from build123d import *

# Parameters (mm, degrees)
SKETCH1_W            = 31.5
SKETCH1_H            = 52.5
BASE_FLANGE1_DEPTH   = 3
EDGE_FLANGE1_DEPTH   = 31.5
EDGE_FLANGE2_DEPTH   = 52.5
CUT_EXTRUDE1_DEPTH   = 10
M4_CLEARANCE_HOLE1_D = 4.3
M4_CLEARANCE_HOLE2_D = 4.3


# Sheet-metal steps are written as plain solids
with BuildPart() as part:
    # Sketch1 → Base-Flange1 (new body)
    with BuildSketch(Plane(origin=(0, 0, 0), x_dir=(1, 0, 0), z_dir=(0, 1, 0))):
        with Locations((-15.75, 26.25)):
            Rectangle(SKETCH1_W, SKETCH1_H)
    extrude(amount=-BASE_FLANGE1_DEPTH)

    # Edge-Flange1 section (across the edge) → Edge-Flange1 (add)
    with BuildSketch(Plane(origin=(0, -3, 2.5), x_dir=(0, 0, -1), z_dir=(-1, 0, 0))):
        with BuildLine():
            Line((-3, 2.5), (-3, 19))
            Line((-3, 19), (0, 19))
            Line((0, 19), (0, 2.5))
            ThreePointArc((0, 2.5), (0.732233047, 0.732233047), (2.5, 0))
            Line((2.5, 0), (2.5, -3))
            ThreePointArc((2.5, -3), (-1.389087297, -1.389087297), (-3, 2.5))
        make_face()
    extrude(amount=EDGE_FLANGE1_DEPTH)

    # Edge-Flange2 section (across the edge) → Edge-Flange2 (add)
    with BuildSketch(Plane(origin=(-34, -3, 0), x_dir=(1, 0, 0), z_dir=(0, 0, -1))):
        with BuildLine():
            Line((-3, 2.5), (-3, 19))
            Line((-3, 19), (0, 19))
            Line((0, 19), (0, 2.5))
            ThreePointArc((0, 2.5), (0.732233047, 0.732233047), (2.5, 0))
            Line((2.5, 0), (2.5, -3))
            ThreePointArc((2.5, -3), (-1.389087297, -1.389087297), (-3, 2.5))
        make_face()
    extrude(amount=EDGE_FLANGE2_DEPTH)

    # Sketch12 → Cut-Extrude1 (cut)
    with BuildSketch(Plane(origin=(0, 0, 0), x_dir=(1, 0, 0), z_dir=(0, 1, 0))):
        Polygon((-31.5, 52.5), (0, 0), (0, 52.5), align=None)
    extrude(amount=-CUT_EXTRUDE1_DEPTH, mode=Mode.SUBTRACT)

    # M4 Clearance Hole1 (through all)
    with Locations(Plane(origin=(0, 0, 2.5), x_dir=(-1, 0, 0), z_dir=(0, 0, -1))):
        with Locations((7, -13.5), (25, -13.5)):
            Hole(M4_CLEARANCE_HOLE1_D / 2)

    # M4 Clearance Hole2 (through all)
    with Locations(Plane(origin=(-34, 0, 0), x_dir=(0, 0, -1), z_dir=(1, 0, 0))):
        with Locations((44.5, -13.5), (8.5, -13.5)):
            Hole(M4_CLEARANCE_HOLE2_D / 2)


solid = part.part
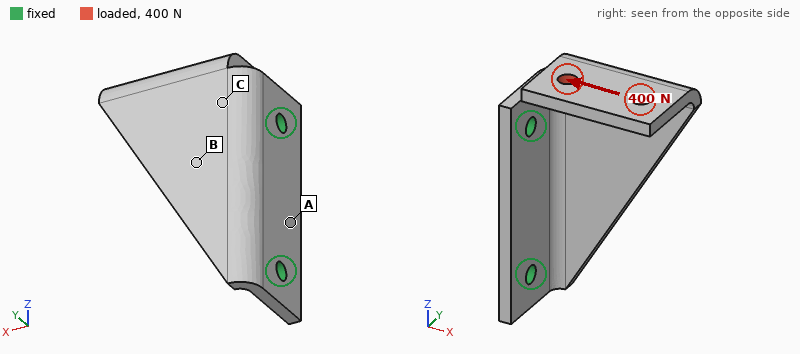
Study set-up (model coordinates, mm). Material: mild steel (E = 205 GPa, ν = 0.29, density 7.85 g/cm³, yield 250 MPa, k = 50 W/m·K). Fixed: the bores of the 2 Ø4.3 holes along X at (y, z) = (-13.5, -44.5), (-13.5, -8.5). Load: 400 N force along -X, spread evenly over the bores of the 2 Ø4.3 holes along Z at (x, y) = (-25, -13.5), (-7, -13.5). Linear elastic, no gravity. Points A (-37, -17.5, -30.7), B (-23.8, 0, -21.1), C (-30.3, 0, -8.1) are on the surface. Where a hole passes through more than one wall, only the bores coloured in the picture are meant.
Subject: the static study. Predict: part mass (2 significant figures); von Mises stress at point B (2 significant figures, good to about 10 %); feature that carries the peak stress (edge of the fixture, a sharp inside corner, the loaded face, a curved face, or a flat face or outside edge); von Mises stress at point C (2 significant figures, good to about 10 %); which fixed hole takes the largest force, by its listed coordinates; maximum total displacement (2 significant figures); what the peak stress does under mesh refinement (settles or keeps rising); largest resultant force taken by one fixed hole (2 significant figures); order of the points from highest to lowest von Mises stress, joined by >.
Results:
63 g
56 MPa
a sharp inside corner
98 MPa
(-13.5, -8.5)
0.23 mm
keeps rising
520 N
C > B > A
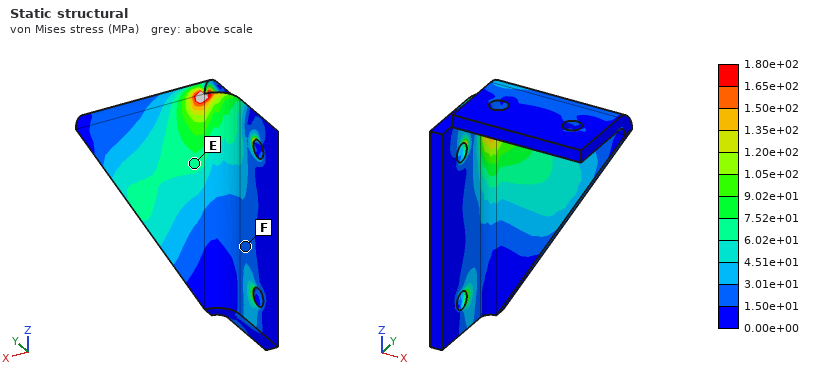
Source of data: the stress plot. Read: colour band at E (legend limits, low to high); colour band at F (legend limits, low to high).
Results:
6.02e+01 to 7.52e+01 MPa
1.50e+01 to 3.01e+01 MPa
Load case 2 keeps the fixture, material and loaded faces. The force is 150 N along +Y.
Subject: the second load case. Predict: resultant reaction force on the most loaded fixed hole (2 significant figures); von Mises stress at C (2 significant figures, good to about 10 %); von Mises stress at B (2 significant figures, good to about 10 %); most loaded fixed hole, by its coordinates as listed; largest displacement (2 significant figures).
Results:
200 N
59 MPa
39 MPa
(-13.5, -8.5)
0.19 mm
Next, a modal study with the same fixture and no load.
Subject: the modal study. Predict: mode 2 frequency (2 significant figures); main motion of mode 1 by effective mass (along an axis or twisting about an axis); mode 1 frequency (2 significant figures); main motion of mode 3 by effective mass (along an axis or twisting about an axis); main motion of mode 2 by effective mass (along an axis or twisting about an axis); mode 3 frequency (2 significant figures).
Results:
2600 Hz
along Y
1200 Hz
along X
along Z
3600 Hz
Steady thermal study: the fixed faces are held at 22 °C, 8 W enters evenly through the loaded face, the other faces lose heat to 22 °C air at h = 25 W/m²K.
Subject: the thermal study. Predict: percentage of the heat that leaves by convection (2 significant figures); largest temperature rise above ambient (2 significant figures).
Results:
41 %
61 K
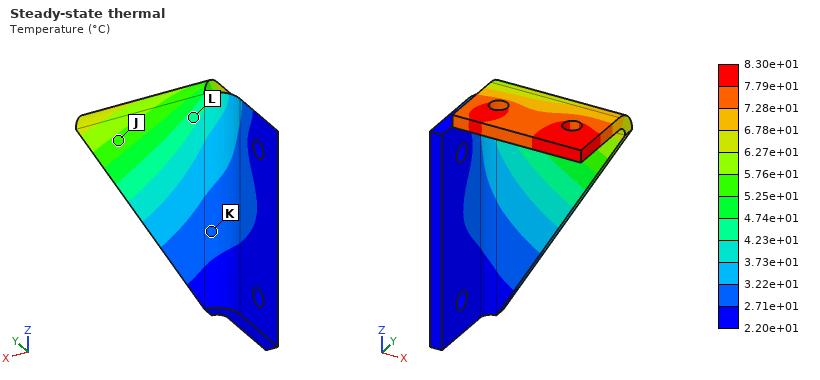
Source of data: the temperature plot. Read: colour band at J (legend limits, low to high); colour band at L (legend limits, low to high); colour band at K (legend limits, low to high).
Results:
5.25e+01 to 5.76e+01 °C
4.23e+01 to 4.74e+01 °C
2.71e+01 to 3.22e+01 °C
